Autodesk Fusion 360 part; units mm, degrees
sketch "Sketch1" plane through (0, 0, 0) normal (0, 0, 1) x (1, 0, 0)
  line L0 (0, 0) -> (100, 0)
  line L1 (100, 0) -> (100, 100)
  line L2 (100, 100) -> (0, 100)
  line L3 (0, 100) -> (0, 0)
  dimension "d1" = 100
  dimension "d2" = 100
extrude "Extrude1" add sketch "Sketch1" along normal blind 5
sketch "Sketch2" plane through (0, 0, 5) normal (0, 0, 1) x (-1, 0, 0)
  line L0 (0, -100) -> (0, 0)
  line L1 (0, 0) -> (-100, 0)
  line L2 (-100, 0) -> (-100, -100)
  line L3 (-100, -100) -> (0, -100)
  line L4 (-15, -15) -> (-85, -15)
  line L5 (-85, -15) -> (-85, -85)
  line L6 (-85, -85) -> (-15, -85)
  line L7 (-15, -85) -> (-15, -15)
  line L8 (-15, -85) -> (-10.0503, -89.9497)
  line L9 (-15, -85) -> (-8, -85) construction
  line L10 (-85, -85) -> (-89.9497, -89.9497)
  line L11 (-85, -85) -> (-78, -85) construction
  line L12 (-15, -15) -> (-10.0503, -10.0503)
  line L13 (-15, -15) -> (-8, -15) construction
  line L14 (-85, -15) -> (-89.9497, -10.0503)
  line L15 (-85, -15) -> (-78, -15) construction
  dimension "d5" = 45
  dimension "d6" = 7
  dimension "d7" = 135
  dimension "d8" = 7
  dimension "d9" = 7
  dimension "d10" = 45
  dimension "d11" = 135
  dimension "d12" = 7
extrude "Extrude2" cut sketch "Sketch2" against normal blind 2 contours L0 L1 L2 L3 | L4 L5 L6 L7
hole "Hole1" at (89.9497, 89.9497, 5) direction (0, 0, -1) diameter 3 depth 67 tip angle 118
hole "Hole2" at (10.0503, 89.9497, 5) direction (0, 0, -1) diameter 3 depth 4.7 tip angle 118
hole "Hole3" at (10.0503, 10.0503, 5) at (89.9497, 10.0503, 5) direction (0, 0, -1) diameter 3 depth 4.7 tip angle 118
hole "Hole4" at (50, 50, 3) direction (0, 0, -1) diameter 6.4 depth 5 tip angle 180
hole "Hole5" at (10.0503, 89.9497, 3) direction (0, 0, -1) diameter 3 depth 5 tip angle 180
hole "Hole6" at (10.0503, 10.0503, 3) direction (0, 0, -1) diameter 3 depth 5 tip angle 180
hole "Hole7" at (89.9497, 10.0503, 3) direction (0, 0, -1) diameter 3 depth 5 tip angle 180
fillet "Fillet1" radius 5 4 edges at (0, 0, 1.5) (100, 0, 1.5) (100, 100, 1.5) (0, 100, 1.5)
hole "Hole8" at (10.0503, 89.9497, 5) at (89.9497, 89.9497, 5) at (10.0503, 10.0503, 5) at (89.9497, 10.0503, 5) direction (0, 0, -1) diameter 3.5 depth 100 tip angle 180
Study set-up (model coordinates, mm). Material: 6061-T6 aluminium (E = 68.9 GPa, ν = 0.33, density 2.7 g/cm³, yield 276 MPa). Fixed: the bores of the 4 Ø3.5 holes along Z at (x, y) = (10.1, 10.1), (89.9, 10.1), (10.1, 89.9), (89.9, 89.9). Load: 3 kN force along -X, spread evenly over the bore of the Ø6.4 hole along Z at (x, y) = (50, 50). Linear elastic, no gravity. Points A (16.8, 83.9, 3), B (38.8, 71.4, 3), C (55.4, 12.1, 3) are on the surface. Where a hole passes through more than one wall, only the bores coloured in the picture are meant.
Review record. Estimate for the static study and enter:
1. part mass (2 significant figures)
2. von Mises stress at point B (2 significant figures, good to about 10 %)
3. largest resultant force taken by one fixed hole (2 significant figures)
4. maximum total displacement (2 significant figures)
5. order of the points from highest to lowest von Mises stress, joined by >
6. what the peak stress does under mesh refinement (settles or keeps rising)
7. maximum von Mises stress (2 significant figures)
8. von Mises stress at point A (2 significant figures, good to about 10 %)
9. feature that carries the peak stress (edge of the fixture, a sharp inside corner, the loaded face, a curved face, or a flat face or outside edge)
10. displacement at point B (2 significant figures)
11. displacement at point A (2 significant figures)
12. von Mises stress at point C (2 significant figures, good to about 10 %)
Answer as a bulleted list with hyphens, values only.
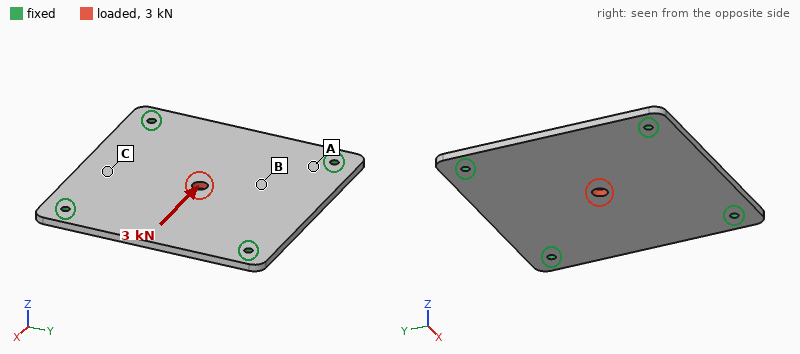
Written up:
- 80 g
- 11 MPa
- 830 N
- 17 µm
- A > B > C
- settles
- 88 MPa
- 16 MPa
- the loaded face
- 7.0 µm
- 2.9 µm
- 4.4 MPa
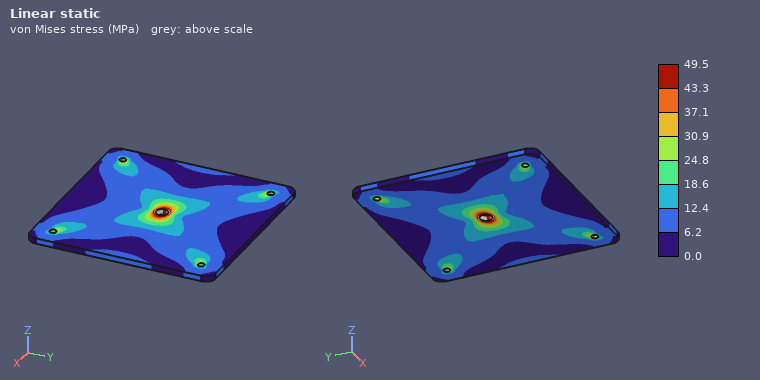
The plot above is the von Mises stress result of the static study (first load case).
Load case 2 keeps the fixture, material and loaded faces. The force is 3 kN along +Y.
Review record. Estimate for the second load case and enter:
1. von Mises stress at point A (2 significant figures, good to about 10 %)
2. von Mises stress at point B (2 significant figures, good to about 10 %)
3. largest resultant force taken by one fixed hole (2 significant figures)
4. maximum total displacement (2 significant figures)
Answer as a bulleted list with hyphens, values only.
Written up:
- 16 MPa
- 11 MPa
- 830 N
- 17 µm
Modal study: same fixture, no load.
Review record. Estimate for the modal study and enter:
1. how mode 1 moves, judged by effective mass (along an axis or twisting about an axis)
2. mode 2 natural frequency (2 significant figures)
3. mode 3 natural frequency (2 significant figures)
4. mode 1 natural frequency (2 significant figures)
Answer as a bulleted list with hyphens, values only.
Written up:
- along Z
- 2600 Hz
- 2600 Hz
- 1600 Hz
